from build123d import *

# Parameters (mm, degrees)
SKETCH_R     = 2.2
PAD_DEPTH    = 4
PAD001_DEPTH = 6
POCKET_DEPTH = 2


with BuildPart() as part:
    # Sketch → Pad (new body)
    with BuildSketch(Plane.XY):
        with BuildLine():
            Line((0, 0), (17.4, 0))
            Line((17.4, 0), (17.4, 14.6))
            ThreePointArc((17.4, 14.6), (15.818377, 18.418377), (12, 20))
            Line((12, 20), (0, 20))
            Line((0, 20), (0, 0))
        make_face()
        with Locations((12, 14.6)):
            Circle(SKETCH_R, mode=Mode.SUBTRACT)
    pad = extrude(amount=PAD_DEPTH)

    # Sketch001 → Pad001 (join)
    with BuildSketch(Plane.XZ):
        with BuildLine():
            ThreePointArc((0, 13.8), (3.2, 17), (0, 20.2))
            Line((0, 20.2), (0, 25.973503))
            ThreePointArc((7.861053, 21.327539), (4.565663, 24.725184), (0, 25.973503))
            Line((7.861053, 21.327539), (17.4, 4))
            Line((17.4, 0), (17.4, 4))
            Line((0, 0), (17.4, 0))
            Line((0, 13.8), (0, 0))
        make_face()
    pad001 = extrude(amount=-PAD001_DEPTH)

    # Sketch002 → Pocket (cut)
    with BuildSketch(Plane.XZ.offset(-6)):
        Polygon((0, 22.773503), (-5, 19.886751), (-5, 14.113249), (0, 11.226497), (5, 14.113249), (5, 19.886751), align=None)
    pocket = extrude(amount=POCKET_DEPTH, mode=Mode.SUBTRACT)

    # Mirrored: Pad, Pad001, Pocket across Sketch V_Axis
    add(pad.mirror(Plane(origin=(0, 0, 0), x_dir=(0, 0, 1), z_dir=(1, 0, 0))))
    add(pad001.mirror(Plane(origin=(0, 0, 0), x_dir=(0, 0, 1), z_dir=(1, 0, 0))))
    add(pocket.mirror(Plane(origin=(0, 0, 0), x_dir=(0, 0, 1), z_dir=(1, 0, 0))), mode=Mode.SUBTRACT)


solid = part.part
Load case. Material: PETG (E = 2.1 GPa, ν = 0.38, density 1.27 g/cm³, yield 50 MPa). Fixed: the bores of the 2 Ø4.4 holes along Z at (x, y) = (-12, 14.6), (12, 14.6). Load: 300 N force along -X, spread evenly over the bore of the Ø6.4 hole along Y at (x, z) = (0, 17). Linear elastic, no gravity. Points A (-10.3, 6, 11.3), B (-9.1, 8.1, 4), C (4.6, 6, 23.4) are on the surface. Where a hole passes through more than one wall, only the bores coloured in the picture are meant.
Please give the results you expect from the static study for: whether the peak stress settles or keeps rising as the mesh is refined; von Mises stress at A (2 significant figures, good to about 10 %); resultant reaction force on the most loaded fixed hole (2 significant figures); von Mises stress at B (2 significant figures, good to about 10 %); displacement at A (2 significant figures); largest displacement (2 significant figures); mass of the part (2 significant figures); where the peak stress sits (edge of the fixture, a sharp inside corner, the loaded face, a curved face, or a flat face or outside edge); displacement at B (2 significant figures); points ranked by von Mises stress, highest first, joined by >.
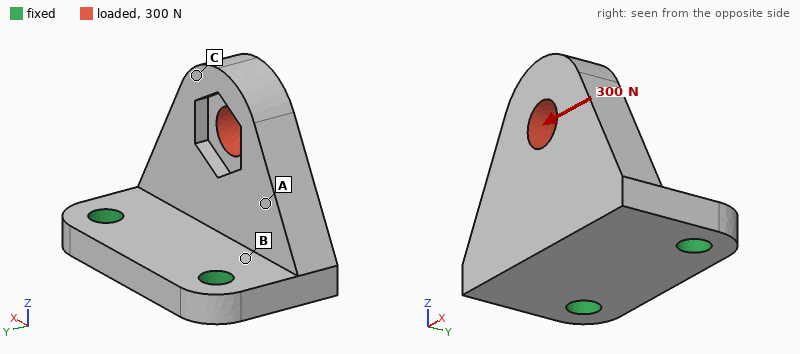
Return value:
keeps rising
7.3 MPa
270 N
13 MPa
0.26 mm
0.47 mm
6.7 g
edge of the fixture
0.081 mm
B > A > C
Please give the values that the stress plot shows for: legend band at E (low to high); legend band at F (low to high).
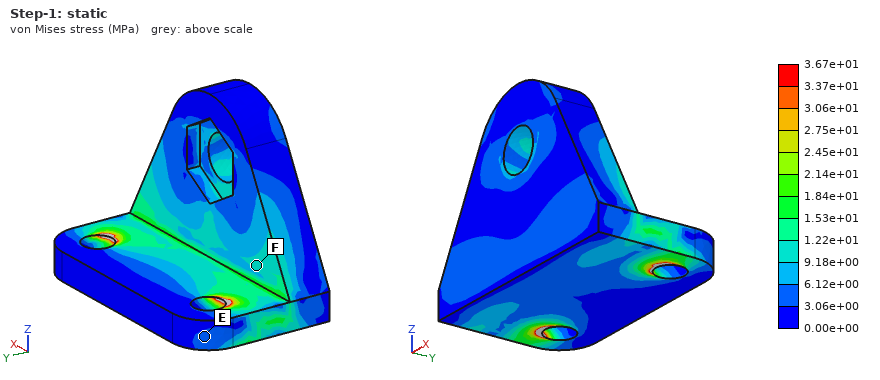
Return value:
3.06e+00 to 6.12e+00 MPa
9.18e+00 to 1.22e+01 MPa
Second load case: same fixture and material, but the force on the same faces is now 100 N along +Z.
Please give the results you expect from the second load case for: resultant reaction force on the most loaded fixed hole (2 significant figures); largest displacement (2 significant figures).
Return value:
50 N
0.51 mm
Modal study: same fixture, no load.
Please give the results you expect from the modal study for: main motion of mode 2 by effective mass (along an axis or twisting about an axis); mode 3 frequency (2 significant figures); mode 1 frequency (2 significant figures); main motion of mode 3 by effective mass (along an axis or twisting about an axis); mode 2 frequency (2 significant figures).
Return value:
along X
3700 Hz
1200 Hz
along Z
2800 Hz
